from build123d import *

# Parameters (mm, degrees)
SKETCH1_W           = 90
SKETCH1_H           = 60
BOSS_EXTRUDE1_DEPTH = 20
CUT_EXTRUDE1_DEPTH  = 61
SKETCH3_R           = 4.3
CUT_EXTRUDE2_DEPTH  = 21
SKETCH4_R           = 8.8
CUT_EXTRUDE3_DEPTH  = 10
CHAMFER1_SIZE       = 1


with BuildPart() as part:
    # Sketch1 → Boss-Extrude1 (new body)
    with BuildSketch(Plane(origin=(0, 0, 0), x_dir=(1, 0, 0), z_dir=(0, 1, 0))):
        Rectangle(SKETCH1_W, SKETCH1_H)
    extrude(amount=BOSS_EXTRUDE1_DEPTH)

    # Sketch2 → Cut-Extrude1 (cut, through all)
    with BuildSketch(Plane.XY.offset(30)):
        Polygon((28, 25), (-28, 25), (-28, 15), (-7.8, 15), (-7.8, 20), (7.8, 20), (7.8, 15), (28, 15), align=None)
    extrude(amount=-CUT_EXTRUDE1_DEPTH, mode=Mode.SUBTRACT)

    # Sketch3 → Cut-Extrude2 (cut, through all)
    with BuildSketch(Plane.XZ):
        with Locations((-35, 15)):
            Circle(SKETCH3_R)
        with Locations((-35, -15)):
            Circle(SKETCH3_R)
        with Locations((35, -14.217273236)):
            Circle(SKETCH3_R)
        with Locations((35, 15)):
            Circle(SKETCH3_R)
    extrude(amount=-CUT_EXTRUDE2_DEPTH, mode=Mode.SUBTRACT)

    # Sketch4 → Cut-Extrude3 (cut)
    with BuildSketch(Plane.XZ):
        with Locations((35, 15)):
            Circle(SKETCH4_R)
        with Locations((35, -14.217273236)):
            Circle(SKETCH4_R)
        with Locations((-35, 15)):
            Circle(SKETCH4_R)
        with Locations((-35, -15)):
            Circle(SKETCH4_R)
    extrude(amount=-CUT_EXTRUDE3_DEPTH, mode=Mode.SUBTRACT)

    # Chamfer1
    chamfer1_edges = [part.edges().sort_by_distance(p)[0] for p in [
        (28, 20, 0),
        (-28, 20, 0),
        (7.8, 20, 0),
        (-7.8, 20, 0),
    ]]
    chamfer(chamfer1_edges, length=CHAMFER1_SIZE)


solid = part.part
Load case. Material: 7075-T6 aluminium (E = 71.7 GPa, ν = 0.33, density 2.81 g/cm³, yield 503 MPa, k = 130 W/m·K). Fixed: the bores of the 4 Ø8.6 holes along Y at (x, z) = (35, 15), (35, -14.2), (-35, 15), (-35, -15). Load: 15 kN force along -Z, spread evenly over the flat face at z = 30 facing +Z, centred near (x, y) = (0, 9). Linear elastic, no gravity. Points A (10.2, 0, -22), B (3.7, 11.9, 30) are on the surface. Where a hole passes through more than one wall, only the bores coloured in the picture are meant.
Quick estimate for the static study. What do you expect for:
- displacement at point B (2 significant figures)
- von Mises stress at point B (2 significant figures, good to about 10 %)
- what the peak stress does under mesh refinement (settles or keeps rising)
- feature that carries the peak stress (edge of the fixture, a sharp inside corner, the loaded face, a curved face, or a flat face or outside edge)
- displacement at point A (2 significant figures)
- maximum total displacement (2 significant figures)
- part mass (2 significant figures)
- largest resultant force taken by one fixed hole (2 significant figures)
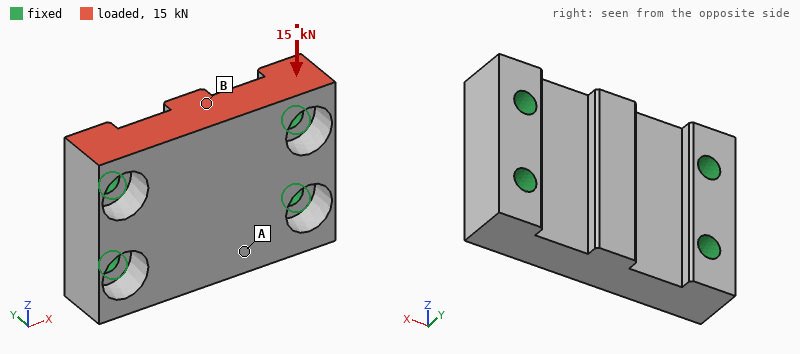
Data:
11 µm
11 MPa
keeps rising
edge of the fixture
7.5 µm
16 µm
240 g
5.2 kN
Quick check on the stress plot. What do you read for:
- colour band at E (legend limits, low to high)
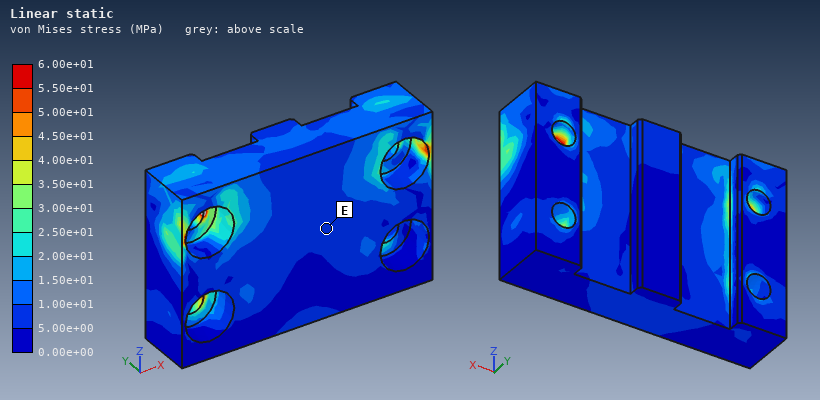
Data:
5.00e+00 to 1.00e+01 MPa
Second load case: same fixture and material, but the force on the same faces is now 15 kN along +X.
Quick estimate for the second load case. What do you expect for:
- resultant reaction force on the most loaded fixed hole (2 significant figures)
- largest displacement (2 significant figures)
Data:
6.6 kN
20 µm
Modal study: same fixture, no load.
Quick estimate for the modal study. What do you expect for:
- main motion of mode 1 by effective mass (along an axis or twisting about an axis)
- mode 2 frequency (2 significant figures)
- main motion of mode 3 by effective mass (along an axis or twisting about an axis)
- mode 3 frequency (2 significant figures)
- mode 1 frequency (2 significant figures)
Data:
along Y
11 kHz
along Z
15 kHz
10 kHz
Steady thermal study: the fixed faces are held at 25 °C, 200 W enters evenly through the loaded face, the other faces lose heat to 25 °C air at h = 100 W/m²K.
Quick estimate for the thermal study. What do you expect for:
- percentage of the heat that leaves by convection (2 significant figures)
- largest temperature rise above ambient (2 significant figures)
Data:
8.2 %
34 K
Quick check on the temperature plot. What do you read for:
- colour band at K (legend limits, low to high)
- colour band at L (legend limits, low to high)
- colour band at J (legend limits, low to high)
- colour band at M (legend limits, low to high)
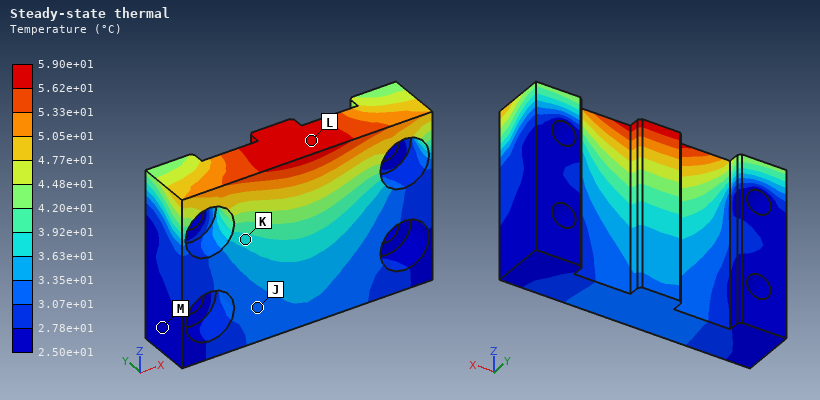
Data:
3.63e+01 to 3.92e+01 °C
5.62e+01 to 5.90e+01 °C
3.07e+01 to 3.35e+01 °C
2.50e+01 to 2.78e+01 °C
